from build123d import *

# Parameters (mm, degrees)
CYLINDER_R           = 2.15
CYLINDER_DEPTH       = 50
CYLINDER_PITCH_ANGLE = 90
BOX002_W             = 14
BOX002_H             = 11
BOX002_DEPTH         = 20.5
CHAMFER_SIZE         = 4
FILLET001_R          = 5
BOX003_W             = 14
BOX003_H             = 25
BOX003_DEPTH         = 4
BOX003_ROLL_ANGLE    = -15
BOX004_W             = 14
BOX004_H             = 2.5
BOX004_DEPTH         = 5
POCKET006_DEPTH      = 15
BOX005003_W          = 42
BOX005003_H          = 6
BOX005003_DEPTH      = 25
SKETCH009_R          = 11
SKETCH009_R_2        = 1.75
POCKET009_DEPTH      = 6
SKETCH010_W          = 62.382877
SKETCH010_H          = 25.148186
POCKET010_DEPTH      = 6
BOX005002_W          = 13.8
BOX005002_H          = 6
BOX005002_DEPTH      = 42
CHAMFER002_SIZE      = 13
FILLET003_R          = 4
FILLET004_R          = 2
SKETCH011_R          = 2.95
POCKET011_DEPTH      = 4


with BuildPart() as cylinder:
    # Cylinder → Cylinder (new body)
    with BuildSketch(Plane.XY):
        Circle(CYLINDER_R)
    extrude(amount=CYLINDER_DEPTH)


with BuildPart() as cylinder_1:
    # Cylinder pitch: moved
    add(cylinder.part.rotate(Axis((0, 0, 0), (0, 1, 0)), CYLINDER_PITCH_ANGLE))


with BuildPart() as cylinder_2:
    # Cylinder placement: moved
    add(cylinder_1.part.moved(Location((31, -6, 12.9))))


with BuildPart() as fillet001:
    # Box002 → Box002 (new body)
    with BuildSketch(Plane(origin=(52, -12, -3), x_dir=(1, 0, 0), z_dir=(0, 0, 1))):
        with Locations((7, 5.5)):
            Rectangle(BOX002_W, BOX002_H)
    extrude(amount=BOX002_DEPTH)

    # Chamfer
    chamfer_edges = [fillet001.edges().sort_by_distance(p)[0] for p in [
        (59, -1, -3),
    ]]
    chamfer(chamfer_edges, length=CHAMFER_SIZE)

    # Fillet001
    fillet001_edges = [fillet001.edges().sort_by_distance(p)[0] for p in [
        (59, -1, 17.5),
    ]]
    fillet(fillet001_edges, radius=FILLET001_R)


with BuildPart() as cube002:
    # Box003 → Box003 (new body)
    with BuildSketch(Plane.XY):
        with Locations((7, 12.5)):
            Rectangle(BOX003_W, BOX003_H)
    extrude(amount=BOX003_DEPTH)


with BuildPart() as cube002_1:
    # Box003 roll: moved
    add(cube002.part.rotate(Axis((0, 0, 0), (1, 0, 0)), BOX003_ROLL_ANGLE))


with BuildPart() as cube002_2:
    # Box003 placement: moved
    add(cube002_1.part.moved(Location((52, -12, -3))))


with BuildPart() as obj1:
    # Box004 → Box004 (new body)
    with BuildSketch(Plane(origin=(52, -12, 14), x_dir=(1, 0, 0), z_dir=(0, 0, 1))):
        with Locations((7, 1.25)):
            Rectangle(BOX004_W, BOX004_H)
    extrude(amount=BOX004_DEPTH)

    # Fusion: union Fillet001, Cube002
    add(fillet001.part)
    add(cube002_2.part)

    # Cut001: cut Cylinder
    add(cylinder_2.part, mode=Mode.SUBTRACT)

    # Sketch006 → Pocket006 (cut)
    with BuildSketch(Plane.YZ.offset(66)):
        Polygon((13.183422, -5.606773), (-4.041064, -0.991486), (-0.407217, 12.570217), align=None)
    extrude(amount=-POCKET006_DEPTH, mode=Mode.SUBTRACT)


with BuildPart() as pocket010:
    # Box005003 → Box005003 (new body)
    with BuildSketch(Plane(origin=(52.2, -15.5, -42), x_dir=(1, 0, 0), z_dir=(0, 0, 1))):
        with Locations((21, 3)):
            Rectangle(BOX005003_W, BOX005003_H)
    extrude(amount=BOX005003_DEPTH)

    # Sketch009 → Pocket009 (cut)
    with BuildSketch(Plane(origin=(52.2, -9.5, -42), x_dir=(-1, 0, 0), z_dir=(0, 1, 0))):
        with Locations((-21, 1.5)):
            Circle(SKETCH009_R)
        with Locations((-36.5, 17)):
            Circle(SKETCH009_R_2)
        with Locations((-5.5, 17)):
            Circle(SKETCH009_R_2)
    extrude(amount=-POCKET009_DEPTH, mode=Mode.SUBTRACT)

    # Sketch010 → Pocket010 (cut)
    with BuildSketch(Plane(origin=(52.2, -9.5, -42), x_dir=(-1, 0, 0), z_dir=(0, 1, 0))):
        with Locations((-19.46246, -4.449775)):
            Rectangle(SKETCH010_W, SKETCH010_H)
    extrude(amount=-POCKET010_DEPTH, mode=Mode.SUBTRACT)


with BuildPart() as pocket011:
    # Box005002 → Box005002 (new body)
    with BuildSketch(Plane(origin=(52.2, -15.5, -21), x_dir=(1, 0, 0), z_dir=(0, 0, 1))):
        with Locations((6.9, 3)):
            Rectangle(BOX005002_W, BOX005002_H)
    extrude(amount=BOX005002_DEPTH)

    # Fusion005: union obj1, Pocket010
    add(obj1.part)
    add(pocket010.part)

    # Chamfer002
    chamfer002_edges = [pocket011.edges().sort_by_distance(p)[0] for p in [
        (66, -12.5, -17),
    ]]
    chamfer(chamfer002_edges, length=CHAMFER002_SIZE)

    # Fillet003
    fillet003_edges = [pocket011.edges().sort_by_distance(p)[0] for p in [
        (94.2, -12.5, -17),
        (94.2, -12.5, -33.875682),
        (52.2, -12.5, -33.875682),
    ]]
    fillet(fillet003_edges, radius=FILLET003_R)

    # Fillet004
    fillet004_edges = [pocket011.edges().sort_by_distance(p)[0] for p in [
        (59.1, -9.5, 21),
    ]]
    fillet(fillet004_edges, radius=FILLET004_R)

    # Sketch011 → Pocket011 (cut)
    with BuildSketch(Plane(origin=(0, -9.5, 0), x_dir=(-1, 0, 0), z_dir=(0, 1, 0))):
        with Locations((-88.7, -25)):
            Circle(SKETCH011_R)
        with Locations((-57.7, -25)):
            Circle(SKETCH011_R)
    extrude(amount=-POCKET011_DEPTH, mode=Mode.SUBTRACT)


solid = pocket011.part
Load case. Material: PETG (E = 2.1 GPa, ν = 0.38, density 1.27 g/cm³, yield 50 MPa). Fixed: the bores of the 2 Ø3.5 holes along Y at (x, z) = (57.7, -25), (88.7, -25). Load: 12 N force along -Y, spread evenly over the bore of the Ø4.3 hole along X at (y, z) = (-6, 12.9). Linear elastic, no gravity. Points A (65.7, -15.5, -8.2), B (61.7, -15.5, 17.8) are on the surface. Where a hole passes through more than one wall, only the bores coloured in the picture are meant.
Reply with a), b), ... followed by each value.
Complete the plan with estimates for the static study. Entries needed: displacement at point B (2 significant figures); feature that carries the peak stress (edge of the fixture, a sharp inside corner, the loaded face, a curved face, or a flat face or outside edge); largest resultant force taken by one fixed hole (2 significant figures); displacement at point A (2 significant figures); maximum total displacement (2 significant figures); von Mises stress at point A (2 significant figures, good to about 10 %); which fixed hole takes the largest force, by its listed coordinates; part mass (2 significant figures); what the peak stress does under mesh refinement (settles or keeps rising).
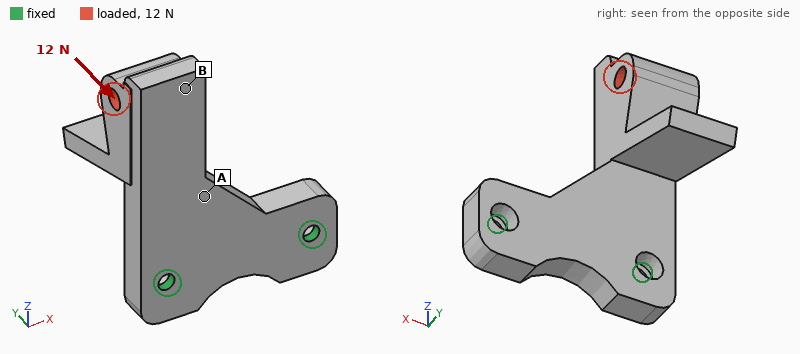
a) 0.69 mm
b) edge of the fixture
c) 13 N
d) 0.20 mm
e) 0.76 mm
f) 3.0 MPa
g) (57.7, -25)
h) 13 g
i) keeps rising
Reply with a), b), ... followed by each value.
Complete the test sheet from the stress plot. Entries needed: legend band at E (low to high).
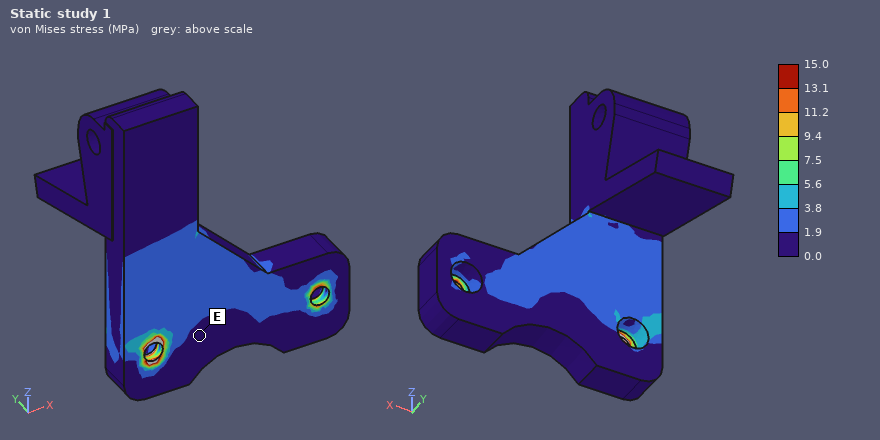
a) 0.0 to 1.9 MPa
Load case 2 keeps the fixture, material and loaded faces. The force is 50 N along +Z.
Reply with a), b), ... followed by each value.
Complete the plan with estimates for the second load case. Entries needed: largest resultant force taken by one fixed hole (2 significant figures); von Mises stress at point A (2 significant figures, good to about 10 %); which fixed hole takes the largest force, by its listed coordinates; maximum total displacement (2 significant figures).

a) 46 N
b) 3.2 MPa
c) (57.7, -25)
d) 0.76 mm
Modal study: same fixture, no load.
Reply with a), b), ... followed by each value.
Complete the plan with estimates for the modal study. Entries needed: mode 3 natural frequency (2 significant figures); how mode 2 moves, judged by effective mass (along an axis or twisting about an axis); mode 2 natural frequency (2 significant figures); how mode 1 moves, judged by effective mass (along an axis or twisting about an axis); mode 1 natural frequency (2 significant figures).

a) 1500 Hz
b) along X
c) 1100 Hz
d) along Y
e) 330 Hz
